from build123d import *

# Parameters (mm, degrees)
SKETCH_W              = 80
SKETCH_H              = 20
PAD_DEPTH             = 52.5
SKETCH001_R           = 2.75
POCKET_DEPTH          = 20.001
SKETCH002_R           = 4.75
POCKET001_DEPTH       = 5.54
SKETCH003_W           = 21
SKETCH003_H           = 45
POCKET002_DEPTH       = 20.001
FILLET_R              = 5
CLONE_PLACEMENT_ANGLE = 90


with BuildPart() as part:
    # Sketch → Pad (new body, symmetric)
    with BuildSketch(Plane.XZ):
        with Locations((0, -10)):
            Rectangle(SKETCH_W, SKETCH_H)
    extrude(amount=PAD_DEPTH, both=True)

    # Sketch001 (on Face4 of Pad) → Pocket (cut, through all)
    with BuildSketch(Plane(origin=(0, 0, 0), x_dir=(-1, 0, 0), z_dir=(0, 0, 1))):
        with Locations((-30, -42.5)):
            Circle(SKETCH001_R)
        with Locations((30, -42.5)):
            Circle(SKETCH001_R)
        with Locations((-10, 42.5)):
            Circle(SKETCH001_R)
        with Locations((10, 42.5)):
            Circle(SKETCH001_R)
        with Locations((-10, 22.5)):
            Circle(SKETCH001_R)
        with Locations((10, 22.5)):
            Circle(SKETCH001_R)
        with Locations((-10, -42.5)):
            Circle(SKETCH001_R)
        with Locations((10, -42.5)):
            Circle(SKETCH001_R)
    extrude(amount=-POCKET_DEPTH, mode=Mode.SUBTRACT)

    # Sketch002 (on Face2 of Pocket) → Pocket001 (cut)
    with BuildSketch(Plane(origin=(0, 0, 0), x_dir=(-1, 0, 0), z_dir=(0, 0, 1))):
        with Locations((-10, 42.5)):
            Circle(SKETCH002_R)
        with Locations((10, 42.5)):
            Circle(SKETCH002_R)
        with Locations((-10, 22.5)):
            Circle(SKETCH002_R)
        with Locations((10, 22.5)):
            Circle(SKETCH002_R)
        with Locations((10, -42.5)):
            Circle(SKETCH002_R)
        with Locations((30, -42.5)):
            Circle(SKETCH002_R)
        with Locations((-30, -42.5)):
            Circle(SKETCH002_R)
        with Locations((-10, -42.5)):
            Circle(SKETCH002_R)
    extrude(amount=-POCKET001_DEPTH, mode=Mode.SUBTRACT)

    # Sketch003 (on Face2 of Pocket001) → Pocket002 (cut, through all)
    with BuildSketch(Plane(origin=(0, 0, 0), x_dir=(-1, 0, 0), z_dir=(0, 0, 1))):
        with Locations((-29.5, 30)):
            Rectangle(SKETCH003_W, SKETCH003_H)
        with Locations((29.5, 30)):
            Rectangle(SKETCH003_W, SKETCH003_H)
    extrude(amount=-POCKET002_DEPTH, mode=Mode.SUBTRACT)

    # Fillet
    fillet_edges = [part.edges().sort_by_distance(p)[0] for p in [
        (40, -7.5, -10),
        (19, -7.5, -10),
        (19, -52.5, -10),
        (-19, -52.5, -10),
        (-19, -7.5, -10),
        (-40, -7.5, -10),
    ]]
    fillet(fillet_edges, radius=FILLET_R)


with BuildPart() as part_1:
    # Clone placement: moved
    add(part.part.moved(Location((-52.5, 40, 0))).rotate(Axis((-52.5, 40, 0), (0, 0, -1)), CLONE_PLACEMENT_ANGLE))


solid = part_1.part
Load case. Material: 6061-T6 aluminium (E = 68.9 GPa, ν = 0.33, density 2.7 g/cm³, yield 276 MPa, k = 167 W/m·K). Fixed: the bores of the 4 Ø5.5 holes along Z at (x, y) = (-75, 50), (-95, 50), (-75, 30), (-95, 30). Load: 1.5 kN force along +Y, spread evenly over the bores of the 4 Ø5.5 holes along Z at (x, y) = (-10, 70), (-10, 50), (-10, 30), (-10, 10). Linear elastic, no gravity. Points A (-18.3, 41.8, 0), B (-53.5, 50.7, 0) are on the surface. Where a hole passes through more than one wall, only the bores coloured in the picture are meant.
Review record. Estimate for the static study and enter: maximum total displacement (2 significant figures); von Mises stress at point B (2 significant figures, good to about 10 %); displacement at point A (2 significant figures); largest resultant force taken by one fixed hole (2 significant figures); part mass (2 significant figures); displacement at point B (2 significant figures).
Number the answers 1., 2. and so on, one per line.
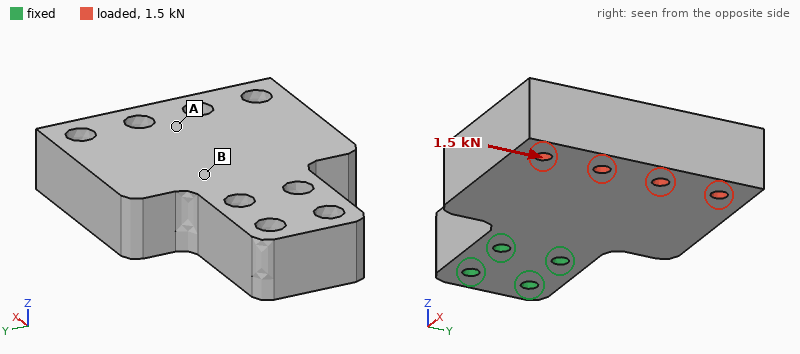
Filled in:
1. 37 µm
2. 6.1 MPa
3. 22 µm
4. 3.4 kN
5. 340 g
6. 7.1 µm
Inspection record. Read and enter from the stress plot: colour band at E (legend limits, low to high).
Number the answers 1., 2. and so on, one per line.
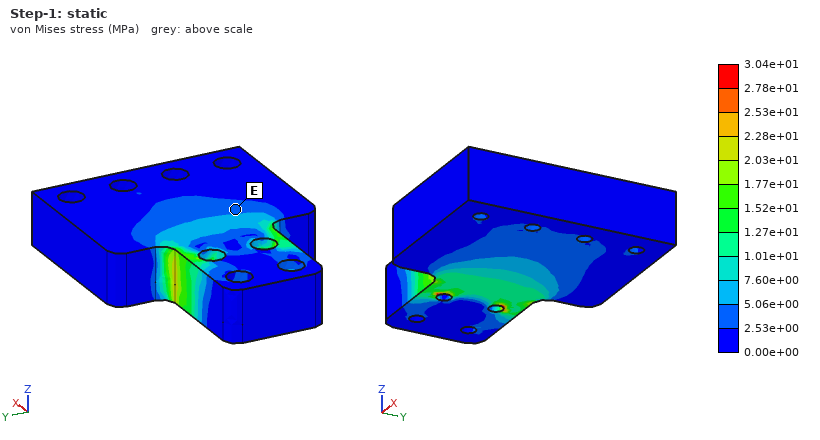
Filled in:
1. 2.53e+00 to 5.06e+00 MPa
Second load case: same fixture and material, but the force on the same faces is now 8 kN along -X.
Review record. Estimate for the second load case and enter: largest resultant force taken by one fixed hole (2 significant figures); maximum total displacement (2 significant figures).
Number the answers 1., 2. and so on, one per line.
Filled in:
1. 3.5 kN
2. 26 µm
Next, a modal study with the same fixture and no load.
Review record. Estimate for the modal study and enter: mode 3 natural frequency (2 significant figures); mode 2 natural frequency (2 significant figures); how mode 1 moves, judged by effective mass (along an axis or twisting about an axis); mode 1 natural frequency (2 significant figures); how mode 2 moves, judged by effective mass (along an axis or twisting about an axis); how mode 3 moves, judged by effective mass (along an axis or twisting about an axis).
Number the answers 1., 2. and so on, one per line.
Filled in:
1. 3500 Hz
2. 3000 Hz
3. along Z
4. 1900 Hz
5. along Y
6. twisting about X
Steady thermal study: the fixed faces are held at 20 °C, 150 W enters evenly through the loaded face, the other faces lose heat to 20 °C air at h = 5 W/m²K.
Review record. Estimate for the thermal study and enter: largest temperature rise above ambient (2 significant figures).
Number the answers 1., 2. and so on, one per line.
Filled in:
1. 56 K
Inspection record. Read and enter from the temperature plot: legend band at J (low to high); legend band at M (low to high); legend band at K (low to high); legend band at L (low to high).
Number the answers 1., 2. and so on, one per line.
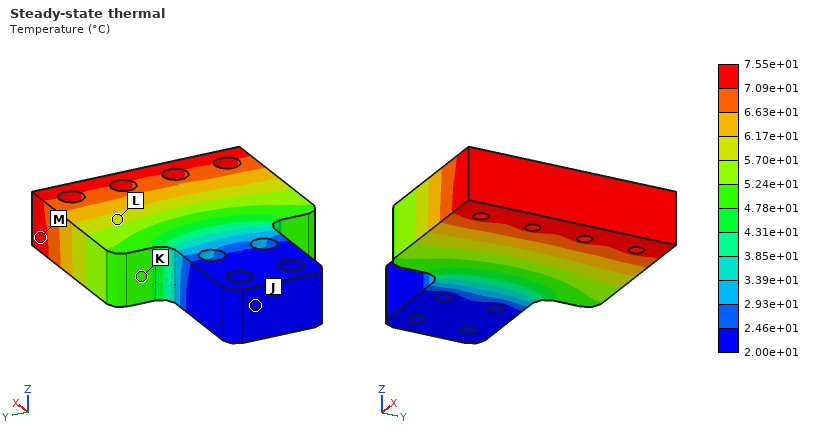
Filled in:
1. 2.00e+01 to 2.46e+01 °C
2. 7.09e+01 to 7.55e+01 °C
3. 4.78e+01 to 5.24e+01 °C
4. 5.70e+01 to 6.17e+01 °C
